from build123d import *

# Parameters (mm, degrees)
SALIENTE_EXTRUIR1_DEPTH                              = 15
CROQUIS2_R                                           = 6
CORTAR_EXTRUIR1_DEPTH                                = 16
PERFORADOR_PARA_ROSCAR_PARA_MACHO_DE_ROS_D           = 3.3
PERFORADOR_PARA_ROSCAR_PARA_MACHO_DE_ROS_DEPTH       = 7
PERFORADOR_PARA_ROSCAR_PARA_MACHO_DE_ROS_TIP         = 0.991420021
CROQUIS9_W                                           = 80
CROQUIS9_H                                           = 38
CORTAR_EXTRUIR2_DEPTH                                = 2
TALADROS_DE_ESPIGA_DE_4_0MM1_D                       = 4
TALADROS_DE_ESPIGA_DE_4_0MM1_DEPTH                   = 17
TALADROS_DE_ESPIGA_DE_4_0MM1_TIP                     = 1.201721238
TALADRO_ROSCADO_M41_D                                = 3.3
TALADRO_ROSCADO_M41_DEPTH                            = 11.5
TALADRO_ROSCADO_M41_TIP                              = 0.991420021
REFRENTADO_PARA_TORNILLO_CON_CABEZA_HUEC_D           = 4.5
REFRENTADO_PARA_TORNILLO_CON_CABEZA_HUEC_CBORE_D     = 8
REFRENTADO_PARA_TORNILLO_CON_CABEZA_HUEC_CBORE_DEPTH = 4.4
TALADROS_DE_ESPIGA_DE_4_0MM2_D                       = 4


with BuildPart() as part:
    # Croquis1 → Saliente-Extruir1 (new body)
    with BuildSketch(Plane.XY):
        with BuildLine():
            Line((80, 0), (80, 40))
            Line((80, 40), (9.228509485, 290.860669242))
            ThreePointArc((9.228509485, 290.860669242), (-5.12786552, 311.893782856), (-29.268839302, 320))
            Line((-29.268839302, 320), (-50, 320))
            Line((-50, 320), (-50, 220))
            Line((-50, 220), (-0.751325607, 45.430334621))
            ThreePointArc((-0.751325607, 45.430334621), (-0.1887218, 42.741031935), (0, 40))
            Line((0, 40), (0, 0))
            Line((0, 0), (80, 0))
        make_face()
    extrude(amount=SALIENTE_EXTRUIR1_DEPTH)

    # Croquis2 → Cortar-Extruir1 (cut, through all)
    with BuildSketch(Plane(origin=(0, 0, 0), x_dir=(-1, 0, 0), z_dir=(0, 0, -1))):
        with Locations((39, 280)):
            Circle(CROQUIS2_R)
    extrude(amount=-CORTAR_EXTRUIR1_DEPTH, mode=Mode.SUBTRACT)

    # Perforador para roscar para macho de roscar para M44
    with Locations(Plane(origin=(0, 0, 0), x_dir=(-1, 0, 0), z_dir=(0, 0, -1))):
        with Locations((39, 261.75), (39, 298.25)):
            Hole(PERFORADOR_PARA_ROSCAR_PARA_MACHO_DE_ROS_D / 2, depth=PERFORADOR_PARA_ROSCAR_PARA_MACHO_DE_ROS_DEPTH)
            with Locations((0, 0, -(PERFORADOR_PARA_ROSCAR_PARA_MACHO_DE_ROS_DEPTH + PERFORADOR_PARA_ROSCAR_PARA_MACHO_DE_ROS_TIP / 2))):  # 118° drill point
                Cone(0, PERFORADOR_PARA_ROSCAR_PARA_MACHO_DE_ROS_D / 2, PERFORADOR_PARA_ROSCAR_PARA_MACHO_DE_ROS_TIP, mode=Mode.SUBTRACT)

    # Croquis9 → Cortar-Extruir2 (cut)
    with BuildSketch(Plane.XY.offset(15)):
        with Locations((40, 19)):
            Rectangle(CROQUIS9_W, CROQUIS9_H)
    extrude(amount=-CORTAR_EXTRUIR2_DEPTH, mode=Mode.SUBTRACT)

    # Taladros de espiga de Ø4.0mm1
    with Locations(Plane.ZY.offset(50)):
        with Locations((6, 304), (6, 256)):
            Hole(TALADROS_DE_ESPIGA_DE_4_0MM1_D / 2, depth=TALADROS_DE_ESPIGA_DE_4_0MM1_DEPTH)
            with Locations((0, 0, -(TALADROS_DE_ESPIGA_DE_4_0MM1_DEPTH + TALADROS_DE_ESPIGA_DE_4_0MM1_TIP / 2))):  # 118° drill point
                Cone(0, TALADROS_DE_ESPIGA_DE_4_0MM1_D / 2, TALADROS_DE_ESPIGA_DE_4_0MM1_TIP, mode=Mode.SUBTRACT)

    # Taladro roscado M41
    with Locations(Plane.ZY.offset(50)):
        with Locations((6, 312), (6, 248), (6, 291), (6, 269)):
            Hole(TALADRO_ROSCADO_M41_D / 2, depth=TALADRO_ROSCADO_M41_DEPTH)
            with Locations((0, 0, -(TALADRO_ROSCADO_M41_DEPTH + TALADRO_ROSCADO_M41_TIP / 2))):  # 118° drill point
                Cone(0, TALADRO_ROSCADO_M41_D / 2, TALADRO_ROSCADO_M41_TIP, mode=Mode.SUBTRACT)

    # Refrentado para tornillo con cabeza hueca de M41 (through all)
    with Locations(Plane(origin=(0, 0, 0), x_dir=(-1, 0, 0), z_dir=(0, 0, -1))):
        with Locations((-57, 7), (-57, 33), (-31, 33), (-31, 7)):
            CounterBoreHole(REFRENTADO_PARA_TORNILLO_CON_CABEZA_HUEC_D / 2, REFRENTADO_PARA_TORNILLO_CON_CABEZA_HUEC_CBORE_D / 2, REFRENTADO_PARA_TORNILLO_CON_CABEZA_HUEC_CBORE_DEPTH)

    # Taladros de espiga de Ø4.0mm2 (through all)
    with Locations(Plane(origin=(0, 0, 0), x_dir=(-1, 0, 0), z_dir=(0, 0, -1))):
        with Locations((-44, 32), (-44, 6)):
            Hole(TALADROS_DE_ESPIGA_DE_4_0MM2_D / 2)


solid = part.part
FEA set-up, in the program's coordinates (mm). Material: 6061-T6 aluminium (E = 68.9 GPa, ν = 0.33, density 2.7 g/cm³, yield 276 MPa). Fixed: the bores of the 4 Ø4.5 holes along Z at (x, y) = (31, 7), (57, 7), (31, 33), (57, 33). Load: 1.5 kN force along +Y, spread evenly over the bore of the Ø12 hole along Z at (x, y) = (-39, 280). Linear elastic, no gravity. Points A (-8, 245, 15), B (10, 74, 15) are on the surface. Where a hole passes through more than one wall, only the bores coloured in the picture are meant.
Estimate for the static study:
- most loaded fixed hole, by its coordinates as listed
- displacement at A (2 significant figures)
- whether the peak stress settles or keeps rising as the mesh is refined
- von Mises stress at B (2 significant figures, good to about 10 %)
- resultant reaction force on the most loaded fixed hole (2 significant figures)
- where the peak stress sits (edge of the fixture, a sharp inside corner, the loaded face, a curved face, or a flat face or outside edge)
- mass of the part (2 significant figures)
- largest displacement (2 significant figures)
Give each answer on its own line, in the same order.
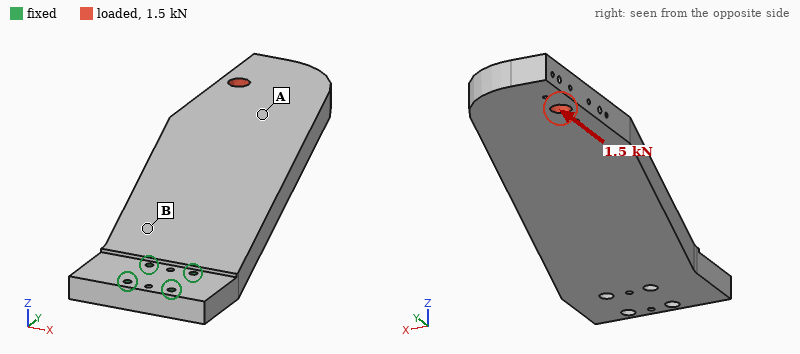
(31, 33)
0.087 mm
keeps rising
5.0 MPa
2.6 kN
edge of the fixture
940 g
0.14 mm
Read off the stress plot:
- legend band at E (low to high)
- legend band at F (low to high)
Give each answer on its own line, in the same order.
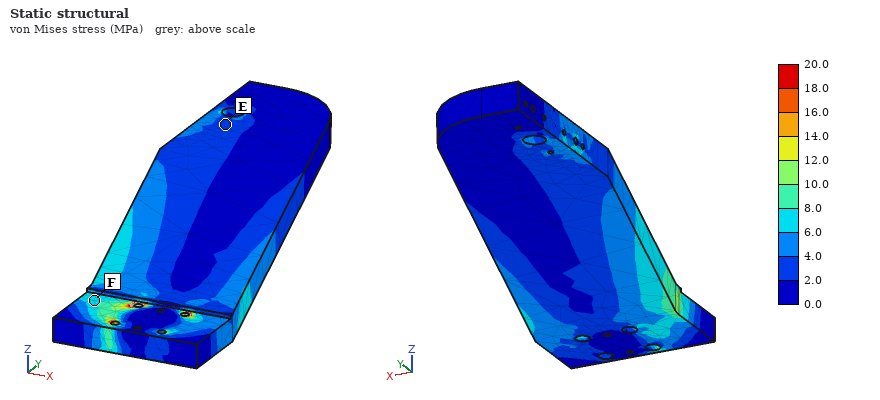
2.0 to 4.0 MPa
6.0 to 8.0 MPa
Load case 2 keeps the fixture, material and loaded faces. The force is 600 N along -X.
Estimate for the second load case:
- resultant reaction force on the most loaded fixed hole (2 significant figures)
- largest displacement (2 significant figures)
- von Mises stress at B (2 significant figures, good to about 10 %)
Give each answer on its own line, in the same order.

2.8 kN
0.16 mm
4.2 MPa
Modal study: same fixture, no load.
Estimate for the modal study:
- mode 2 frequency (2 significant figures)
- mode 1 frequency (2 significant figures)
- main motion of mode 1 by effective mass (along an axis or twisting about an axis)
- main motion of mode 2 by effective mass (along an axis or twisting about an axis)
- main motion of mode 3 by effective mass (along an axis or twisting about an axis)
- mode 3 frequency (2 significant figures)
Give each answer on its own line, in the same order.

620 Hz
140 Hz
along Z
along X
along Z
860 Hz
